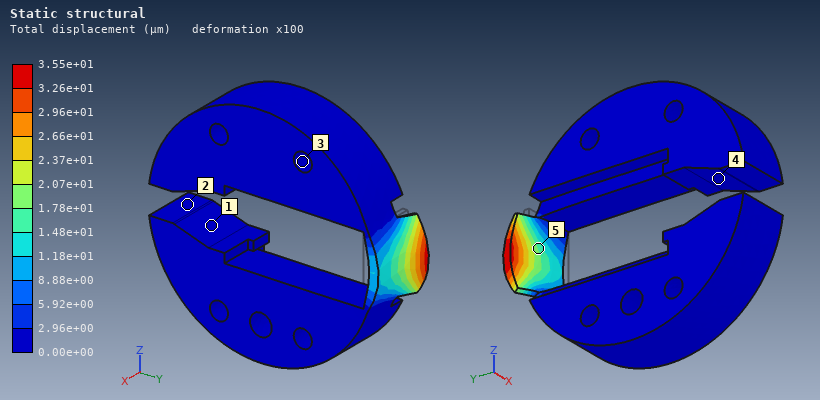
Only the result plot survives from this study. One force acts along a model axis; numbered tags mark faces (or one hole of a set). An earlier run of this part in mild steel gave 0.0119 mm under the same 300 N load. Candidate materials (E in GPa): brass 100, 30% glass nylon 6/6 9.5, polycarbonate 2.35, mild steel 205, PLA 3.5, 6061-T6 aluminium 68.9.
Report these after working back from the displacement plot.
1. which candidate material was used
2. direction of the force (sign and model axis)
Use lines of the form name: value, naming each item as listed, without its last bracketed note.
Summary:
which candidate material was used: 6061-T6 aluminium
direction of the force: +Y
